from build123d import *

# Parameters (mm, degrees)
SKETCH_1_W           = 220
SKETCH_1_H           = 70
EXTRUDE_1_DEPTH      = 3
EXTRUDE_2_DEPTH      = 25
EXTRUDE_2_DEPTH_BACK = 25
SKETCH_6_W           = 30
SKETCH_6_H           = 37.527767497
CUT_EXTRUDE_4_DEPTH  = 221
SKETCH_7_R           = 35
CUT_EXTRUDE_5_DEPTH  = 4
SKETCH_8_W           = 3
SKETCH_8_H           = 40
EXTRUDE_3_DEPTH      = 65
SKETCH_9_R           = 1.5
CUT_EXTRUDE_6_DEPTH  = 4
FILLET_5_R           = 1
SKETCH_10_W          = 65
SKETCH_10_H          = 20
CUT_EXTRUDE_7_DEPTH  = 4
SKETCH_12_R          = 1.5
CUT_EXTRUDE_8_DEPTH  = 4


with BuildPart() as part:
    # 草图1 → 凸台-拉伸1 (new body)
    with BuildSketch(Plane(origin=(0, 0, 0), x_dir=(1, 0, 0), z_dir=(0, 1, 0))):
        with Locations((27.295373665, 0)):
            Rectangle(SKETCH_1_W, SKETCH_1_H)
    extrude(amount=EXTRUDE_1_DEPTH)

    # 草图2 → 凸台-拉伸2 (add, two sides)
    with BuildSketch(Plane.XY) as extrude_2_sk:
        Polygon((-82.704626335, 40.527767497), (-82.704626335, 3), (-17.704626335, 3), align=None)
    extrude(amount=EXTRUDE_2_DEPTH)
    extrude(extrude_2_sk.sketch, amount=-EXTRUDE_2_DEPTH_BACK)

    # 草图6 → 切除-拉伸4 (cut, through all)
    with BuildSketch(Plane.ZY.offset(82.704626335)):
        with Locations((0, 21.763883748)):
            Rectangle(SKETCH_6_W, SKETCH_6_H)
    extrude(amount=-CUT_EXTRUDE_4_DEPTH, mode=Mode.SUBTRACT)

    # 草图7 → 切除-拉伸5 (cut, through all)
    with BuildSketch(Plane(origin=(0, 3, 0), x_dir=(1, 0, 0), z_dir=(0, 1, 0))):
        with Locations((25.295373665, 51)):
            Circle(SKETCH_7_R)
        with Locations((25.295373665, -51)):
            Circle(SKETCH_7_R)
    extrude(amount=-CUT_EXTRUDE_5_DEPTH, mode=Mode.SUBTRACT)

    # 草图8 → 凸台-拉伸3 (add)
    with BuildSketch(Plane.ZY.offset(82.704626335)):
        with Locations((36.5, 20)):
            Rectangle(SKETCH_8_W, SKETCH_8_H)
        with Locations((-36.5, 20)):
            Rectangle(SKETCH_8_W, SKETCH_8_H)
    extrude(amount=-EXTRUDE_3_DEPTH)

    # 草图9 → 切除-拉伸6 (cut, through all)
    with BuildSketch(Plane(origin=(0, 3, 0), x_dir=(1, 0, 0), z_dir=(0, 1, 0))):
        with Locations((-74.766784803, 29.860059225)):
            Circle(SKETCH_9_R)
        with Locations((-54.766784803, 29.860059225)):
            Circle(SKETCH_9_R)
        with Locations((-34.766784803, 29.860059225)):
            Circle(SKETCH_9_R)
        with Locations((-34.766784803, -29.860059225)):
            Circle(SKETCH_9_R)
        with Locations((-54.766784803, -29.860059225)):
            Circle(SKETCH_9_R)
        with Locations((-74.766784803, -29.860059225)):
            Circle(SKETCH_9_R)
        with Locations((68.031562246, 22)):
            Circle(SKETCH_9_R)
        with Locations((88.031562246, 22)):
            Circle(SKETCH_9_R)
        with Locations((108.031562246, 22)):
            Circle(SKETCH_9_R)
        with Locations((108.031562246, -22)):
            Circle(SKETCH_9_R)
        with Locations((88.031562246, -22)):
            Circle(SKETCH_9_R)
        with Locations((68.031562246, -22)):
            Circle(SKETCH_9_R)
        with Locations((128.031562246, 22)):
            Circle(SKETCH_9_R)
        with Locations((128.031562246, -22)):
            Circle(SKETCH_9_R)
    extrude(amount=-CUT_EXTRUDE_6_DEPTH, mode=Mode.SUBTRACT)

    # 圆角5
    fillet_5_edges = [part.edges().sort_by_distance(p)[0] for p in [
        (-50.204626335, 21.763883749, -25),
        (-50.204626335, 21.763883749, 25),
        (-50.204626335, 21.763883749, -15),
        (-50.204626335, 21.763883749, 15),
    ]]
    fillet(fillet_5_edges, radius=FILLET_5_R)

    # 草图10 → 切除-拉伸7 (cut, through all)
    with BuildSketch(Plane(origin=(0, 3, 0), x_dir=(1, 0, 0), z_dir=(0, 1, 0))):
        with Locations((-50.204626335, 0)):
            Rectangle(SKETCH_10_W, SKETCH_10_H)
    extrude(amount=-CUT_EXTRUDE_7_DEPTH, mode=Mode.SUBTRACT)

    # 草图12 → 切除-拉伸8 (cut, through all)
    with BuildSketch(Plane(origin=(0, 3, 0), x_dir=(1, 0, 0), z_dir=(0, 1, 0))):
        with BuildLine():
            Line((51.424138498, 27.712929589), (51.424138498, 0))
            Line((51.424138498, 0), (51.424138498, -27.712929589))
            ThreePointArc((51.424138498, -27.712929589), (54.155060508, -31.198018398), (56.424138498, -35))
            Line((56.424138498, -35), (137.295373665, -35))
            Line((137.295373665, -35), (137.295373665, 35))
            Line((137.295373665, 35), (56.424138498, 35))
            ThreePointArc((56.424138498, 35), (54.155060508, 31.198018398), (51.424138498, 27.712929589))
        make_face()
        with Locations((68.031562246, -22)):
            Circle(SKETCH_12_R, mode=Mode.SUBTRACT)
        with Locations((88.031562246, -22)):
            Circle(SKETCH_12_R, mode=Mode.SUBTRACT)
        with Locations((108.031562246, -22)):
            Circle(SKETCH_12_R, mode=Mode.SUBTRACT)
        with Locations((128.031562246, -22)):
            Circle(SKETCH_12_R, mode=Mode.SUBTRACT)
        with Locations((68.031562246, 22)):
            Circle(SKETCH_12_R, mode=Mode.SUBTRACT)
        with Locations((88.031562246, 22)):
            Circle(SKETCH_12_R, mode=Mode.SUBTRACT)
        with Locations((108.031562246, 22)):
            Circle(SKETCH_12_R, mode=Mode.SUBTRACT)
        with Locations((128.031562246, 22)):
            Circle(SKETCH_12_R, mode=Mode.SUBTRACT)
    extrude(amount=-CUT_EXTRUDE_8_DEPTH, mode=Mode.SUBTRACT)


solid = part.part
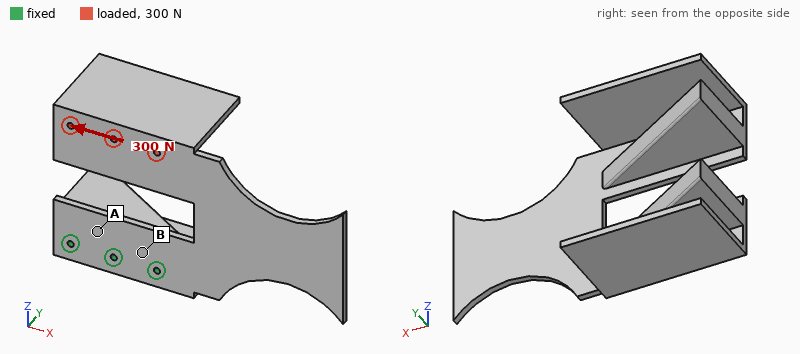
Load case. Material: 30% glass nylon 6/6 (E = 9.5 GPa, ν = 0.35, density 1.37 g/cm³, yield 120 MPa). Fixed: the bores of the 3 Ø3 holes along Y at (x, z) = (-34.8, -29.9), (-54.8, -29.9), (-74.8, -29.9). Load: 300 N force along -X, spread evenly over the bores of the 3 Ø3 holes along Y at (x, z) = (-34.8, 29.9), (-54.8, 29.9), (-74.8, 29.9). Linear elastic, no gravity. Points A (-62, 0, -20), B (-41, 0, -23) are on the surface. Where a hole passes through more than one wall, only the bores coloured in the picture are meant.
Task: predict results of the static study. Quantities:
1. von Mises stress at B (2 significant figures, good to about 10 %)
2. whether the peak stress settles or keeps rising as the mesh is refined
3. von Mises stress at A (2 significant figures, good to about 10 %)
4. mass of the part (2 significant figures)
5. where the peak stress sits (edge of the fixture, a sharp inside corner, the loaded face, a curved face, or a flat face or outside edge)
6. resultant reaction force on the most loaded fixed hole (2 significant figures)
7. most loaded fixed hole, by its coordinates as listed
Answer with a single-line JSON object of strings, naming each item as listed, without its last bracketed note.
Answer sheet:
{"von Mises stress at B": "15 MPa", "whether the peak stress settles or keeps rising as the mesh is refined": "keeps rising", "von Mises stress at A": "6.5 MPa", "mass of the part": "81 g", "where the peak stress sits": "a sharp inside corner", "resultant reaction force on the most loaded fixed hole": "540 N", "most loaded fixed hole, by its coordinates as listed": "(-34.8, -29.9)"}
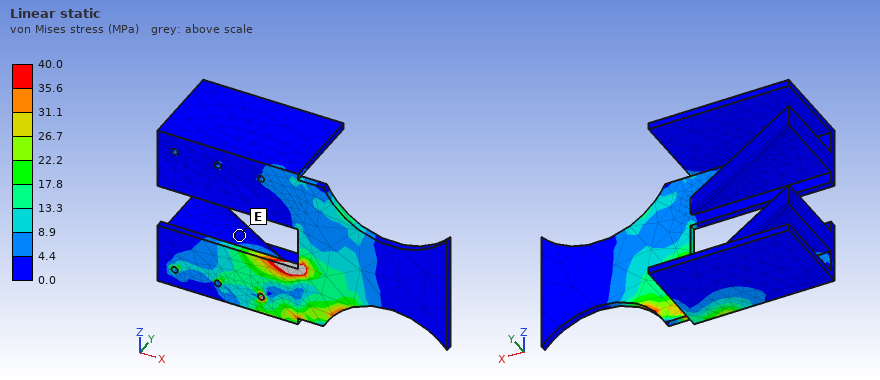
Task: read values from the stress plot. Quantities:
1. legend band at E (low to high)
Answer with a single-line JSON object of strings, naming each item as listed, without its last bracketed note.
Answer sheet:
{"legend band at E": "0.0 to 4.4 MPa"}
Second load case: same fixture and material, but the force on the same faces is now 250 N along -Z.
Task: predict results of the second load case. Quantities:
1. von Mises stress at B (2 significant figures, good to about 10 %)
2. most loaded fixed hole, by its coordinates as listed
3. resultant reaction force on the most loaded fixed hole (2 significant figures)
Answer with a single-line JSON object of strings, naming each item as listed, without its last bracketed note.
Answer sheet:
{"von Mises stress at B": "4.4 MPa", "most loaded fixed hole, by its coordinates as listed": "(-34.8, -29.9)", "resultant reaction force on the most loaded fixed hole": "130 N"}
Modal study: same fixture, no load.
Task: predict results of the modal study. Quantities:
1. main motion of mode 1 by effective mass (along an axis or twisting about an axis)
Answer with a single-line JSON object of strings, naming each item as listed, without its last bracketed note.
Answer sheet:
{"main motion of mode 1 by effective mass": "along Y"}
